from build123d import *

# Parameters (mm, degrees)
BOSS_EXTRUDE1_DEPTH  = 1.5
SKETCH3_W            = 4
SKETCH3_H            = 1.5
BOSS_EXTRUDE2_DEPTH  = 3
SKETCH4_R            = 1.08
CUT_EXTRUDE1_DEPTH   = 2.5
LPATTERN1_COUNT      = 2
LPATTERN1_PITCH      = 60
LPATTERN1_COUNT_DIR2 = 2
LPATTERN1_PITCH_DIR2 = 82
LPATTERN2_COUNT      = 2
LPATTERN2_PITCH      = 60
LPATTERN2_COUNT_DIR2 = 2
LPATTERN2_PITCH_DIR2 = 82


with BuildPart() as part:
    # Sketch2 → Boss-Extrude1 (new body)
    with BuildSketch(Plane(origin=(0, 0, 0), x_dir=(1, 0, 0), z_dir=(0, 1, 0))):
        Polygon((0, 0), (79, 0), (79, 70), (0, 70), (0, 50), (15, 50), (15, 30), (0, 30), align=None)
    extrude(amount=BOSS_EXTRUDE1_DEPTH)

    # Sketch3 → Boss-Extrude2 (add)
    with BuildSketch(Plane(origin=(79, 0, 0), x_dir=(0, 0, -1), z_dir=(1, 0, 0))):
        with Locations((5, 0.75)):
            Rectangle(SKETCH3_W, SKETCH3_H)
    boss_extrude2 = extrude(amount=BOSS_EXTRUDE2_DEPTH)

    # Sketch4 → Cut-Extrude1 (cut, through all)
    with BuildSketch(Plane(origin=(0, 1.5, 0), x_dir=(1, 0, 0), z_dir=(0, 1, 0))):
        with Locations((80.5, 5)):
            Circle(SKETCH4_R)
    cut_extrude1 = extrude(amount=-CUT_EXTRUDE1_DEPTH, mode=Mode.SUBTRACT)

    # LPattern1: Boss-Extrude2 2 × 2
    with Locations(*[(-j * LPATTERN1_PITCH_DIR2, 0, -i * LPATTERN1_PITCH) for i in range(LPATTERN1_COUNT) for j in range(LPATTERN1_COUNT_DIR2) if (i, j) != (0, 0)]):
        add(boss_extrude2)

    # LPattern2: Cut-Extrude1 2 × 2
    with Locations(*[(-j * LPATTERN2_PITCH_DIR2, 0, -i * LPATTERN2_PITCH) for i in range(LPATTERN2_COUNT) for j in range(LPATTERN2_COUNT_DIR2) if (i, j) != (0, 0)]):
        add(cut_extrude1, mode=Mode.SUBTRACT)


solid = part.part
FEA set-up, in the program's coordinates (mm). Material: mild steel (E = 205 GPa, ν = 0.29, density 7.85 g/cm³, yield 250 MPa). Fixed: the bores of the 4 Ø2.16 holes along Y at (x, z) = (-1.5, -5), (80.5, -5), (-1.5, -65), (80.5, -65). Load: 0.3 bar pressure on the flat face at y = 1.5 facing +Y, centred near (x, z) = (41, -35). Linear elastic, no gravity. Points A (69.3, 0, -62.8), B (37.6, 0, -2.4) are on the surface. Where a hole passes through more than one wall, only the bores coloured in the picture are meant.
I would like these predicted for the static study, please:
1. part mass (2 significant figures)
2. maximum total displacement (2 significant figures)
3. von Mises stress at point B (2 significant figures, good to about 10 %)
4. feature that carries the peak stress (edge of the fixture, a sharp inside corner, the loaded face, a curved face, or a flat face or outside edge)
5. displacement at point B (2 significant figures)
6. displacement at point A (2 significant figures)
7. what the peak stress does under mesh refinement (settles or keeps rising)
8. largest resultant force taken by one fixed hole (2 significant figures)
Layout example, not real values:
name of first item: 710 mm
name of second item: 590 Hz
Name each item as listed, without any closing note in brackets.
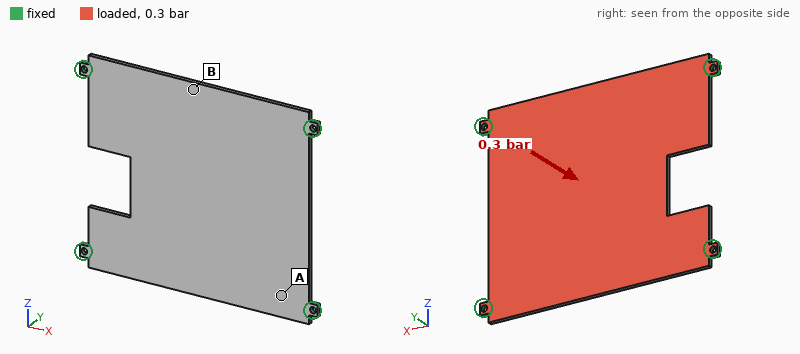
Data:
part mass: 62 g
maximum total displacement: 0.15 mm
von Mises stress at point B: 38 MPa
feature that carries the peak stress: edge of the fixture
displacement at point B: 0.12 mm
displacement at point A: 0.040 mm
what the peak stress does under mesh refinement: keeps rising
largest resultant force taken by one fixed hole: 41 N
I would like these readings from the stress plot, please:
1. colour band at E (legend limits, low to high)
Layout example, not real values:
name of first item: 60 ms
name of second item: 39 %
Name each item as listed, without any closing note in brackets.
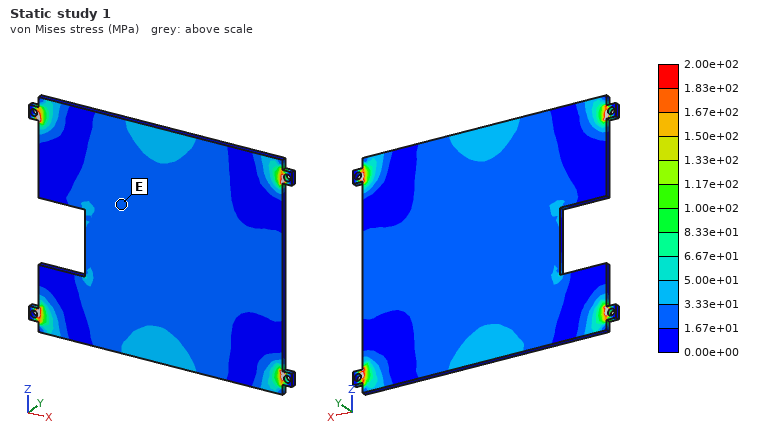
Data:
colour band at E: 1.67e+01 to 3.33e+01 MPa
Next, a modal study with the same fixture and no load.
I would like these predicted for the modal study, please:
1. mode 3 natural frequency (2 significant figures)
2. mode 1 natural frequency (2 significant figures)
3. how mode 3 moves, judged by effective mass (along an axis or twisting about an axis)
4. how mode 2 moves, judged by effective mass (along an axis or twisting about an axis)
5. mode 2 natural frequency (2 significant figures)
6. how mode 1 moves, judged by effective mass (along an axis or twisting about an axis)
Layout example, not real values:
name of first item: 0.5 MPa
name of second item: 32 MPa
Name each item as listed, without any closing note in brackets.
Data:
mode 3 natural frequency: 1800 Hz
mode 1 natural frequency: 760 Hz
how mode 3 moves, judged by effective mass: twisting about Z
how mode 2 moves, judged by effective mass: twisting about X
mode 2 natural frequency: 1300 Hz
how mode 1 moves, judged by effective mass: along Y
